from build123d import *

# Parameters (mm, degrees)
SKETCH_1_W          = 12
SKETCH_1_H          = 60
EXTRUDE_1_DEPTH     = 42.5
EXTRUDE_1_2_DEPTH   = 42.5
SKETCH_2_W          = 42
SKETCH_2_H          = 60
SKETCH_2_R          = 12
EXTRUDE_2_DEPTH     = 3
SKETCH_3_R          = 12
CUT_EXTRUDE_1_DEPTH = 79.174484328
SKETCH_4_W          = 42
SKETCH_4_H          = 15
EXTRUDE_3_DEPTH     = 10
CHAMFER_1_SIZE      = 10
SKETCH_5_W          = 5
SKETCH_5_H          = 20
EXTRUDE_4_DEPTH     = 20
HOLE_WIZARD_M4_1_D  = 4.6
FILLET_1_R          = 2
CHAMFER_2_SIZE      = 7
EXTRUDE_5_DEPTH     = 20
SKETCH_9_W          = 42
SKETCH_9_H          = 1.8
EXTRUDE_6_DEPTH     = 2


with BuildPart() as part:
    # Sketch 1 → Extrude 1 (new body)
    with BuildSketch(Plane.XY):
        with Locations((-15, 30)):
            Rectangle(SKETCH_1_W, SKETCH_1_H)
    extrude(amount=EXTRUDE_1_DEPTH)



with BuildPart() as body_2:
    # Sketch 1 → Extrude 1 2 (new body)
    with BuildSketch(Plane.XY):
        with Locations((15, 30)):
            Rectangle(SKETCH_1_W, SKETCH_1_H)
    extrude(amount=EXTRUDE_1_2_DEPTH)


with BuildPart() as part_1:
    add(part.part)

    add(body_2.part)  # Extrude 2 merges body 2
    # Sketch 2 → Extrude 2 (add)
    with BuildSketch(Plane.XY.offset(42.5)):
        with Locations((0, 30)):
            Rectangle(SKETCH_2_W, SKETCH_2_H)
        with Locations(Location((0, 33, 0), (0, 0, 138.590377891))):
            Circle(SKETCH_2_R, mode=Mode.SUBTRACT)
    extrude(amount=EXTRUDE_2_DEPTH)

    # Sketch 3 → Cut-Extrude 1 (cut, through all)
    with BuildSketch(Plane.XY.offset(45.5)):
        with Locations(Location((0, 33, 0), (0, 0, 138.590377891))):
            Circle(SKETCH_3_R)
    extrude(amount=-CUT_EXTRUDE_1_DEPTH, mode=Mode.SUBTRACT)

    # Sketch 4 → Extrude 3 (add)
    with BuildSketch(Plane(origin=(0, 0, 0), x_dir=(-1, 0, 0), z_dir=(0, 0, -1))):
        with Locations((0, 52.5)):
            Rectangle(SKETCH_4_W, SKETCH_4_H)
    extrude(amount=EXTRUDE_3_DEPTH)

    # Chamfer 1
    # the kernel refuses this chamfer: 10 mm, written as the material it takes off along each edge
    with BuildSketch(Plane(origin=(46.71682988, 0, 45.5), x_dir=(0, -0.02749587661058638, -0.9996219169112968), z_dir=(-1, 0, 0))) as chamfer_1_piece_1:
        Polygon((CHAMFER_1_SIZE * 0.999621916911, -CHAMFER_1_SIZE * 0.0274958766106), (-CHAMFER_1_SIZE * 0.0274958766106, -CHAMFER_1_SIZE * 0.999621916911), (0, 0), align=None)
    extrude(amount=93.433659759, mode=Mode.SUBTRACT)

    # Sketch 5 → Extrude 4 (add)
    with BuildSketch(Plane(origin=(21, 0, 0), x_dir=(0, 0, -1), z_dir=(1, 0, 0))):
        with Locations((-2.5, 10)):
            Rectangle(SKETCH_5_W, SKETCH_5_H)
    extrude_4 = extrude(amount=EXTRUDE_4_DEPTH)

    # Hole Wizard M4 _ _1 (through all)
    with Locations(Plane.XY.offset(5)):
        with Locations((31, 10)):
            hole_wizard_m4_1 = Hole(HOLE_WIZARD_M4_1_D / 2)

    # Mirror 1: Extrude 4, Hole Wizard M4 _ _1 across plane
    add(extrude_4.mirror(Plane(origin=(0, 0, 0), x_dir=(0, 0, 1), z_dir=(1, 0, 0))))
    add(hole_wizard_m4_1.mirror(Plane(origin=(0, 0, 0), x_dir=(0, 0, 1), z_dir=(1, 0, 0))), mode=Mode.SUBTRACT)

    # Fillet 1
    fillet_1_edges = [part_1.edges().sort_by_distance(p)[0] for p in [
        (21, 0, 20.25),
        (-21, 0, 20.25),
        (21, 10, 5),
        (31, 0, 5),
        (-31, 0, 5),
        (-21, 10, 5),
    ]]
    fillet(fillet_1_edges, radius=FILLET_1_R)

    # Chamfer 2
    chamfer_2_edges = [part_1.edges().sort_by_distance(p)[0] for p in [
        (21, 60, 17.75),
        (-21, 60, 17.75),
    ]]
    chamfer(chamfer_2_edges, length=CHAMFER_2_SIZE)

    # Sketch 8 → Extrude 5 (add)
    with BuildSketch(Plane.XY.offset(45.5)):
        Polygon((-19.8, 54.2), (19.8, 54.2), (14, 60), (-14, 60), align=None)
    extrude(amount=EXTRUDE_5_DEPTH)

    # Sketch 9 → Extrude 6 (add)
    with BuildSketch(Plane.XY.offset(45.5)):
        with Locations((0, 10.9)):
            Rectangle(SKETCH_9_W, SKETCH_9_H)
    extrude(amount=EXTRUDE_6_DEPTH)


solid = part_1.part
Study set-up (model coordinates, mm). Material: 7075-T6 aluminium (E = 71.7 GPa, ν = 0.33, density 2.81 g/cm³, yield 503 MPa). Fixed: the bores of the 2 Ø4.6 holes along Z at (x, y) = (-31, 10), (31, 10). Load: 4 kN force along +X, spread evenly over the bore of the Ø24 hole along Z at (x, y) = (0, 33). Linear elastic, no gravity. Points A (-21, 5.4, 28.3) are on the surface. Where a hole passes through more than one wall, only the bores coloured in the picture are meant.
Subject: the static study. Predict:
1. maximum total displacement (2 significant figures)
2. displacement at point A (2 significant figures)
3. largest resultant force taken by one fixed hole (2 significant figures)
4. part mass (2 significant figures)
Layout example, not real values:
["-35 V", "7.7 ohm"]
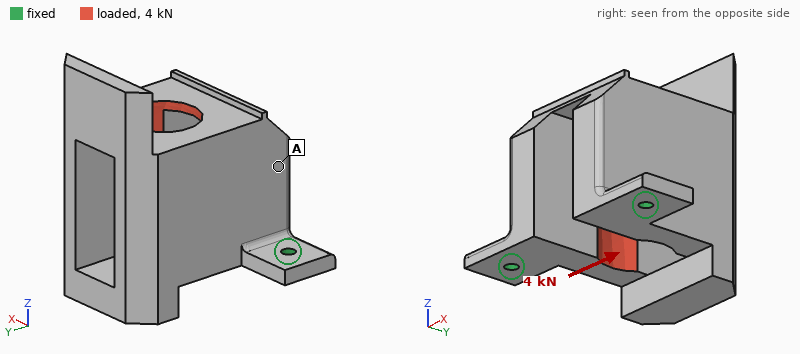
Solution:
["0.15 mm", "0.078 mm", "2.9 kN", "210 g"]
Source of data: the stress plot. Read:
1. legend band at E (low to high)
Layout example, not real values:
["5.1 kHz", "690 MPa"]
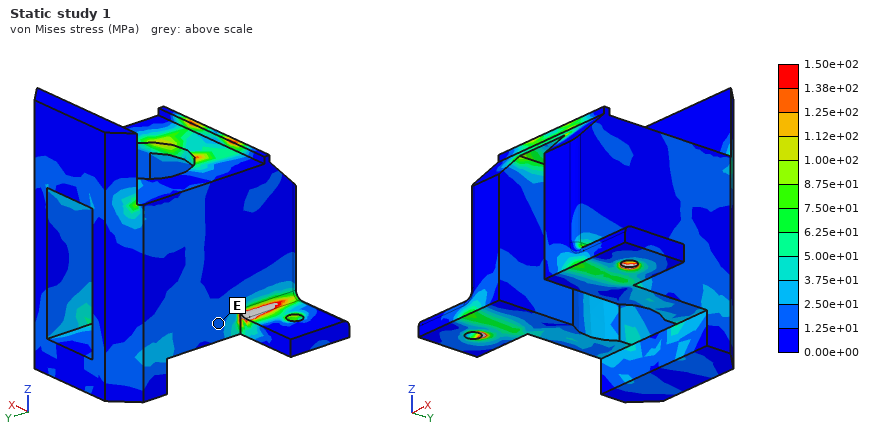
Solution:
["1.25e+01 to 2.50e+01 MPa"]
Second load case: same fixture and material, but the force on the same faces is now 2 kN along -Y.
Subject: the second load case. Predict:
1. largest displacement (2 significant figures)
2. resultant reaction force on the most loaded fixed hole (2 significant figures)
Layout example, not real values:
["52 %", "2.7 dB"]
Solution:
["0.77 mm", "1.0 kN"]
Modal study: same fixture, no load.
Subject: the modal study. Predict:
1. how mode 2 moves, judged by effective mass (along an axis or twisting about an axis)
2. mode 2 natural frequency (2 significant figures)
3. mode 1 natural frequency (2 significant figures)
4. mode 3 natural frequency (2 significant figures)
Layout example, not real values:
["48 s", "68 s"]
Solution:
["along X", "2300 Hz", "620 Hz", "3300 Hz"]
